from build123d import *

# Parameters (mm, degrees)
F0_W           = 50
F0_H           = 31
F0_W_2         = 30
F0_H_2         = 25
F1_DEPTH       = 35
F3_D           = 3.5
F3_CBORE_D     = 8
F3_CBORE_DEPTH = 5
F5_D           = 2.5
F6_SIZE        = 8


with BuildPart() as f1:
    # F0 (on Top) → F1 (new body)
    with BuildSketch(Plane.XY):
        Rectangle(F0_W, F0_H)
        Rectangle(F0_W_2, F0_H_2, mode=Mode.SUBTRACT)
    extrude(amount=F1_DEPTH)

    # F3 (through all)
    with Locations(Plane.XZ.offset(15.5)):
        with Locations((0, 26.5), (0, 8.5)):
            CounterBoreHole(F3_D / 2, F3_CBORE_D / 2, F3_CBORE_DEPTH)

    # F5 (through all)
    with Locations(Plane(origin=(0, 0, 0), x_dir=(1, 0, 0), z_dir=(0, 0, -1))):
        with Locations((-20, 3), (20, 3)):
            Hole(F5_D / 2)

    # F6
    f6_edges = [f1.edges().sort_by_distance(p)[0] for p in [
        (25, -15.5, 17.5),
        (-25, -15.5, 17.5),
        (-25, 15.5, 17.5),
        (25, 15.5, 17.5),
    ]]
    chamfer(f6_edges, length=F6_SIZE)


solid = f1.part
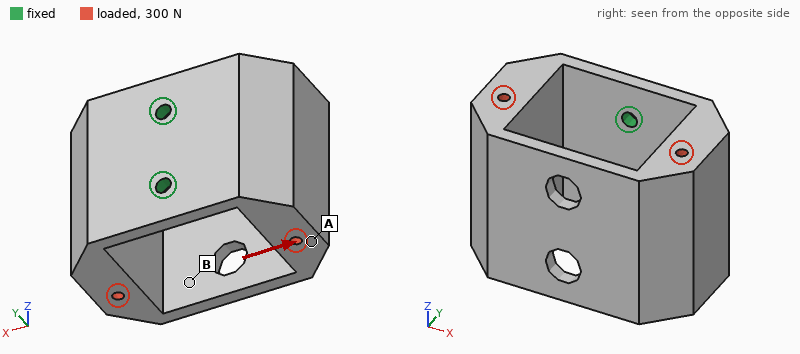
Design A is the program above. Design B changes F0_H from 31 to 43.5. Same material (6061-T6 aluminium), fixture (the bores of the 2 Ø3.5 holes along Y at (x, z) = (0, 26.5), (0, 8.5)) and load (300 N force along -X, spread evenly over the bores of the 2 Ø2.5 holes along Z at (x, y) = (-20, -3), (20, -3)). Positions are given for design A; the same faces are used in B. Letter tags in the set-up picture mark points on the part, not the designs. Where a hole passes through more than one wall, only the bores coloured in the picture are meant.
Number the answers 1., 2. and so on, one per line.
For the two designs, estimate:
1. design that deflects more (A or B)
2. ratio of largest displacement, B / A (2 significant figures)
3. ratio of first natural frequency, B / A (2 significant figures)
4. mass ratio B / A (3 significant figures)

1. A
2. 0.089
3. 2.5
4. 1.93
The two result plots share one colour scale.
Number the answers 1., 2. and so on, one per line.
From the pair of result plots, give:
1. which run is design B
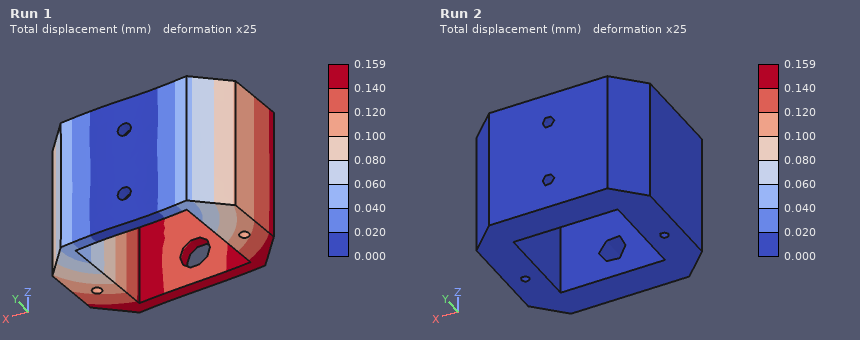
1. Run 2
